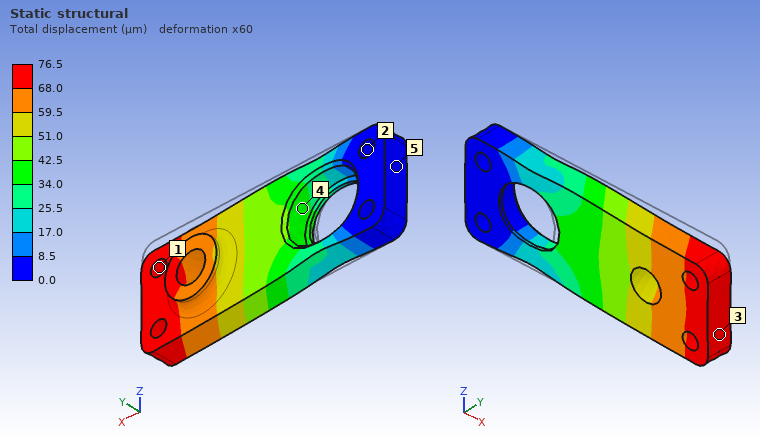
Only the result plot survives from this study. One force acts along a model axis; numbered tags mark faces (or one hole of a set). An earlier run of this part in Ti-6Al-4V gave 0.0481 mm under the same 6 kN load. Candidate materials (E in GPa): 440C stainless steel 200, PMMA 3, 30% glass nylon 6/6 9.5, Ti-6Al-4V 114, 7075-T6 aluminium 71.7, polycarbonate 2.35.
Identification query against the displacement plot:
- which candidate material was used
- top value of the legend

7075-T6 aluminium
76.5 µm
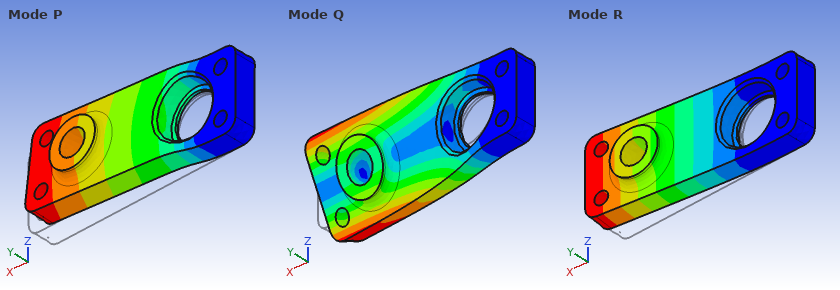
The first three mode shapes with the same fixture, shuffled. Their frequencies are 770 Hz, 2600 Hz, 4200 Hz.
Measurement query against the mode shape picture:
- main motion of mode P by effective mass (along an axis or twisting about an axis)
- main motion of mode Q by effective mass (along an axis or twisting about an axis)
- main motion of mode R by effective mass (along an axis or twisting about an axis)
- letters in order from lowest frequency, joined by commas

along Z
twisting about X
along Y
R, P, Q
